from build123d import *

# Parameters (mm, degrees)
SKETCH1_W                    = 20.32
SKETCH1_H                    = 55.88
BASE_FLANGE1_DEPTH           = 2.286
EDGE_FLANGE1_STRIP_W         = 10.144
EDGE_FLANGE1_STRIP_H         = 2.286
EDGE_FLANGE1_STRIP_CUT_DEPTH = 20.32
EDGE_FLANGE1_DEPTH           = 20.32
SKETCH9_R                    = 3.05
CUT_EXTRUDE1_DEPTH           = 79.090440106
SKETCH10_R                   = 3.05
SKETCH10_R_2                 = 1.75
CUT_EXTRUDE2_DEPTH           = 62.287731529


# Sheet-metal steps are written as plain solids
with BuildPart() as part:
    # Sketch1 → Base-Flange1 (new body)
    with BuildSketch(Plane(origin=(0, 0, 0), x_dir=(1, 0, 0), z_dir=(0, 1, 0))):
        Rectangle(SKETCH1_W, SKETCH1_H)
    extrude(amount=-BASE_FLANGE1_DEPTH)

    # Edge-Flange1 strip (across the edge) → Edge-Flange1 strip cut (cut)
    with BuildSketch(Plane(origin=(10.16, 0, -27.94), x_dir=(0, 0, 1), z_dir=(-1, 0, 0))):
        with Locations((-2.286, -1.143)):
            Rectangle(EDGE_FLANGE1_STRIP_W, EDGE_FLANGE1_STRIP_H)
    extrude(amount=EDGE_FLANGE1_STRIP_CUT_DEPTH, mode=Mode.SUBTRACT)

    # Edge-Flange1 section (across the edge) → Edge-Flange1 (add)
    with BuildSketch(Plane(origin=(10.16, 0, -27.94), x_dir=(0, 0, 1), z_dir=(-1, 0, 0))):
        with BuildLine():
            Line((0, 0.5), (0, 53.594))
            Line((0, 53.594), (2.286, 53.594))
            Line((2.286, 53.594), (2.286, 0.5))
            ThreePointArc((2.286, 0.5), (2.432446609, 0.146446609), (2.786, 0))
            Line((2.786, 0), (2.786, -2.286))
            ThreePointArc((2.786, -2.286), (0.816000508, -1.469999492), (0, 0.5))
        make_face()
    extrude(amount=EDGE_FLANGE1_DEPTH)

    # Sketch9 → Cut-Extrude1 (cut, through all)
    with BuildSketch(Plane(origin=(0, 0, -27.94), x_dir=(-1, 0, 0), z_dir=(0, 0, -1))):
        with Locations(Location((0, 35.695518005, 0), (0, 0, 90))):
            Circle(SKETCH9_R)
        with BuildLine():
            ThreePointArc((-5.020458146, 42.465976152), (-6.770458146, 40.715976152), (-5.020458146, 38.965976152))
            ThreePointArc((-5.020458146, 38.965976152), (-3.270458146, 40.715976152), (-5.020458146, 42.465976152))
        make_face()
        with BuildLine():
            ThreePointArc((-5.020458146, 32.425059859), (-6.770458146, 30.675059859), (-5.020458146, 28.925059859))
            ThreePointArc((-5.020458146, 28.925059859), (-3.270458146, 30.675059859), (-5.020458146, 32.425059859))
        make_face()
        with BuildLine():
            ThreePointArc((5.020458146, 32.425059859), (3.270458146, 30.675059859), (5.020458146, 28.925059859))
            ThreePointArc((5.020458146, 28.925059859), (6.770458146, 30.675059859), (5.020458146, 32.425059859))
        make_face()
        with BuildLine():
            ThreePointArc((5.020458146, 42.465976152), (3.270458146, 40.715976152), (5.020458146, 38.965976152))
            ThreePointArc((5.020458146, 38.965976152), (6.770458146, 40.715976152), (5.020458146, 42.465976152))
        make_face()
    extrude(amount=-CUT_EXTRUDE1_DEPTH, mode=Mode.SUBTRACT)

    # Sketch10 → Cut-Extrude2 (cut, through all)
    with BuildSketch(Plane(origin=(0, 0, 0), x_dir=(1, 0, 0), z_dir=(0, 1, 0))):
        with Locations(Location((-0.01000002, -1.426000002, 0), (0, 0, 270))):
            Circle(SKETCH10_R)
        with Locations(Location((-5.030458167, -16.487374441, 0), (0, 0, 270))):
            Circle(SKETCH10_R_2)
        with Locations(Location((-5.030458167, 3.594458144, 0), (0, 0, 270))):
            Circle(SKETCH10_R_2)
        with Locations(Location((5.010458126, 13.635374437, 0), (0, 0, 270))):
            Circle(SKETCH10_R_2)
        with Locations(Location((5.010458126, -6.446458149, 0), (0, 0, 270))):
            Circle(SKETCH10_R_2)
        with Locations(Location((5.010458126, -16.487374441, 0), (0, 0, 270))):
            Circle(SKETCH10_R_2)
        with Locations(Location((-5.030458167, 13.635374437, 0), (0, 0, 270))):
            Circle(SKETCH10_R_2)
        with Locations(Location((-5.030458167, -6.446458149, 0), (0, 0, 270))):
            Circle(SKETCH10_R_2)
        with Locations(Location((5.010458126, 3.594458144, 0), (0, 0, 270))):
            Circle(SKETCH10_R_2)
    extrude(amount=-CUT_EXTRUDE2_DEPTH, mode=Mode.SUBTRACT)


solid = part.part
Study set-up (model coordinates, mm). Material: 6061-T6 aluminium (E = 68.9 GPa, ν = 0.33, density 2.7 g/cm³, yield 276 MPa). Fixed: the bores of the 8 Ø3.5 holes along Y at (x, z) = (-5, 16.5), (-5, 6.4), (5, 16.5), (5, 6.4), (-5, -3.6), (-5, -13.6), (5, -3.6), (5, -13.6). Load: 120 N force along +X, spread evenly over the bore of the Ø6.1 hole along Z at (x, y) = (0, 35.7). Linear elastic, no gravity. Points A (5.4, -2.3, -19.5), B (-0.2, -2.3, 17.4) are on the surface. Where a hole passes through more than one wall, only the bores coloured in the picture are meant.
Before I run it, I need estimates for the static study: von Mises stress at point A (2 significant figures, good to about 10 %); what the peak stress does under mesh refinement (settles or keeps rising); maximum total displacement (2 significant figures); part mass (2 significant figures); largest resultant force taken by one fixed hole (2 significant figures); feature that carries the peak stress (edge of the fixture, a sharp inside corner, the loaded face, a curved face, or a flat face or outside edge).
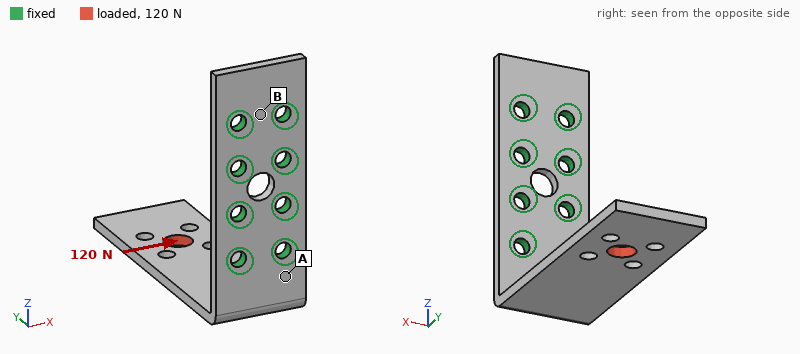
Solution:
120 MPa
keeps rising
0.80 mm
13 g
370 N
edge of the fixture
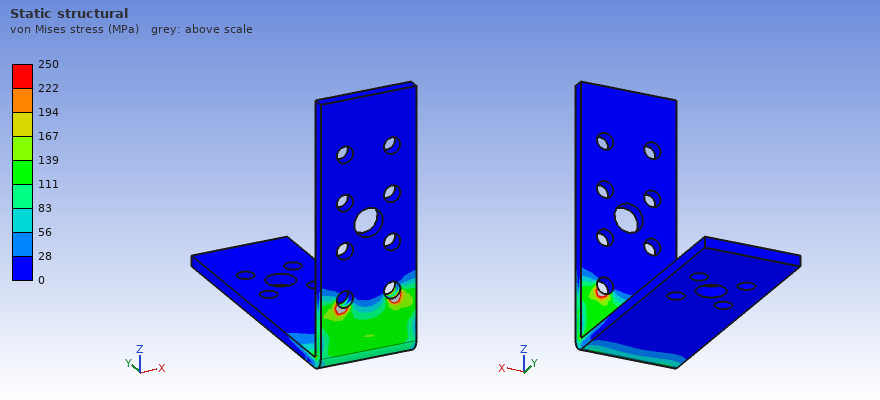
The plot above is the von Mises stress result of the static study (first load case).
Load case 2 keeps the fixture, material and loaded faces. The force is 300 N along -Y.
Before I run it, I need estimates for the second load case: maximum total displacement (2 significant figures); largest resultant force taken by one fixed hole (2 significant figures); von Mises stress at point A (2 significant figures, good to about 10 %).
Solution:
0.85 mm
170 N
110 MPa
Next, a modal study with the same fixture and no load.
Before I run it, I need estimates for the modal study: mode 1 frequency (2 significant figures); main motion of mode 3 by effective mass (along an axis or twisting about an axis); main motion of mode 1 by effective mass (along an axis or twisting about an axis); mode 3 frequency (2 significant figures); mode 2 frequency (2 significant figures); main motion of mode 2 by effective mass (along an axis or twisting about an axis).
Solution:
480 Hz
along Y
along Z
2700 Hz
1100 Hz
along X
